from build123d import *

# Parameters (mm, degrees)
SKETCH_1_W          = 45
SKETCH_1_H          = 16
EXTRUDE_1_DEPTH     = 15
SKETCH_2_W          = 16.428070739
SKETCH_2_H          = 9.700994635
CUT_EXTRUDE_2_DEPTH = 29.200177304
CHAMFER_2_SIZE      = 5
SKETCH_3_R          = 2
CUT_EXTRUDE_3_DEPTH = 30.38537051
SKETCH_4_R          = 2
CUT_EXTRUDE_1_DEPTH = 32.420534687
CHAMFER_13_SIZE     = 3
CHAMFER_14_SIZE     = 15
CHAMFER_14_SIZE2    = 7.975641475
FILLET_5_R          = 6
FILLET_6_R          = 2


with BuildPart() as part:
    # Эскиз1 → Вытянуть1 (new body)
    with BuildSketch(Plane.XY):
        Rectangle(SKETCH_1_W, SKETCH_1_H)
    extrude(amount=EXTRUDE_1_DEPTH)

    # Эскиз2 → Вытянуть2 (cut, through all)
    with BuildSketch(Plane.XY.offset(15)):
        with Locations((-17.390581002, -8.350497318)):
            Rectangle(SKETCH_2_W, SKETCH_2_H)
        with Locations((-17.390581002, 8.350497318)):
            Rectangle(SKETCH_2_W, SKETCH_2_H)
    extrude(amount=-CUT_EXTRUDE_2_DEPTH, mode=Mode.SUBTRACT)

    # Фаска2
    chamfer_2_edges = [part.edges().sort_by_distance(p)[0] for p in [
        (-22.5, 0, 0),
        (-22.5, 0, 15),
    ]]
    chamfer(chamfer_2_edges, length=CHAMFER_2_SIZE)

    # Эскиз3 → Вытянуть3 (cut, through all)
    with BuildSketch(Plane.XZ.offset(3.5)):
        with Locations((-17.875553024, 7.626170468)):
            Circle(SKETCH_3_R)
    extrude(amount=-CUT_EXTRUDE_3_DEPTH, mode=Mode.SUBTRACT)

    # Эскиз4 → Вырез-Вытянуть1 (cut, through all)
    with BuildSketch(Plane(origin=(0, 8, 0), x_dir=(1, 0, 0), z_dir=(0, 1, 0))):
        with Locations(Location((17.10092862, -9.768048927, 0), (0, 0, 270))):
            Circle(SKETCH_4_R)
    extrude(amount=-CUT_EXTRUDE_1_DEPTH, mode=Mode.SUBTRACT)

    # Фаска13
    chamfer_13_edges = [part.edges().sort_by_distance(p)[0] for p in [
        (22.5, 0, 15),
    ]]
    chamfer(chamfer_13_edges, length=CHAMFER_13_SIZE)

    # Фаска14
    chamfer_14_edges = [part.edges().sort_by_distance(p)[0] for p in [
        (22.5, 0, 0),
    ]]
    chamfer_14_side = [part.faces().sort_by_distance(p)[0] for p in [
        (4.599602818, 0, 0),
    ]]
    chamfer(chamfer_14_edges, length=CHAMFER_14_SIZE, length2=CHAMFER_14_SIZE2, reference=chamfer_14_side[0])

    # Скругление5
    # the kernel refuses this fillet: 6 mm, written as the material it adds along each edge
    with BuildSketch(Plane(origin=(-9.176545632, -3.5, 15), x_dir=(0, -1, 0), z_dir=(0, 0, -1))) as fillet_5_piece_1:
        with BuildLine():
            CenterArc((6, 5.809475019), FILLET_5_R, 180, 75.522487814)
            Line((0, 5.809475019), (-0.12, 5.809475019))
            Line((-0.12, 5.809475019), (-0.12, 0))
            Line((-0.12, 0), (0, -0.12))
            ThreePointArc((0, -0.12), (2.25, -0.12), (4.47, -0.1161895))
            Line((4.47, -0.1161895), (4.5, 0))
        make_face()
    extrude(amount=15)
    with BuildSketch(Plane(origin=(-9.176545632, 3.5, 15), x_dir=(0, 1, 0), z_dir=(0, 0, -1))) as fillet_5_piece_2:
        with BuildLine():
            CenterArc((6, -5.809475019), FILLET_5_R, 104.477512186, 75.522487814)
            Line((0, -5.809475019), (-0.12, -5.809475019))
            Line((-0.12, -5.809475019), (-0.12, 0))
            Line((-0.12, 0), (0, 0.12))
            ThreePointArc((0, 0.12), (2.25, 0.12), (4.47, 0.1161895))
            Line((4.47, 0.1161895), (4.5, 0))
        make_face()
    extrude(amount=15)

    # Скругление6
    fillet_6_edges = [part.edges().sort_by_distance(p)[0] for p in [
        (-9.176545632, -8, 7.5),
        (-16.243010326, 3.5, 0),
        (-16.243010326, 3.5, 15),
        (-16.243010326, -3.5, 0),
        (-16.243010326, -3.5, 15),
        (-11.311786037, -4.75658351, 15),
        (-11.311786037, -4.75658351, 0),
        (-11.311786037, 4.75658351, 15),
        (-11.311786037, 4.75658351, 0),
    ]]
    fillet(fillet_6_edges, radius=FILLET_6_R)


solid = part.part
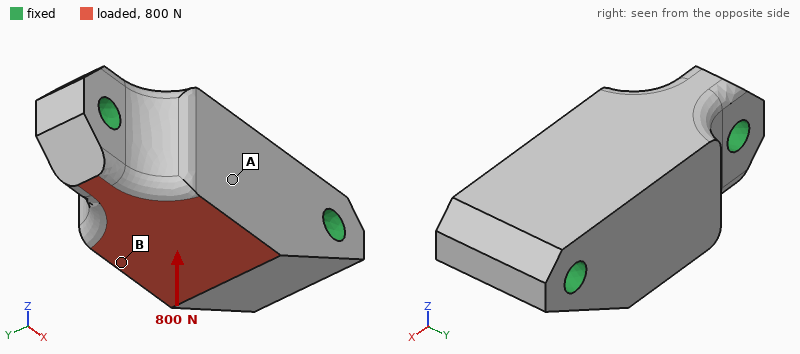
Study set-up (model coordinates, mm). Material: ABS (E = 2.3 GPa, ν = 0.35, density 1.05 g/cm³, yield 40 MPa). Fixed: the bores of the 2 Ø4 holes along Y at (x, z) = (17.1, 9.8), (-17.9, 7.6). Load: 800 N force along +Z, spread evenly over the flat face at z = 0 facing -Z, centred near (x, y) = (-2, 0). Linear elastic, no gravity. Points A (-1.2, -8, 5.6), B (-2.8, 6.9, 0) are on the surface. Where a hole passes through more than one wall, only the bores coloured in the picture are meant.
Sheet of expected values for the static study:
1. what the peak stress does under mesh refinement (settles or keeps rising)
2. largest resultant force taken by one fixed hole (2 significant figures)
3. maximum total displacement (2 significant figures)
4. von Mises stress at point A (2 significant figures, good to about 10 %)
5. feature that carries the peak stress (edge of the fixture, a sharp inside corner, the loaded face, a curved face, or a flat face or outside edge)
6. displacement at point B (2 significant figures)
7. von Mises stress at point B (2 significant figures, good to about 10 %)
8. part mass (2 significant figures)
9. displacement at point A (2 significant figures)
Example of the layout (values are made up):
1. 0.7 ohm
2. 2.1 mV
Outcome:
1. keeps rising
2. 430 N
3. 79 µm
4. 1.7 MPa
5. edge of the fixture
6. 77 µm
7. 5.4 MPa
8. 8.1 g
9. 74 µm
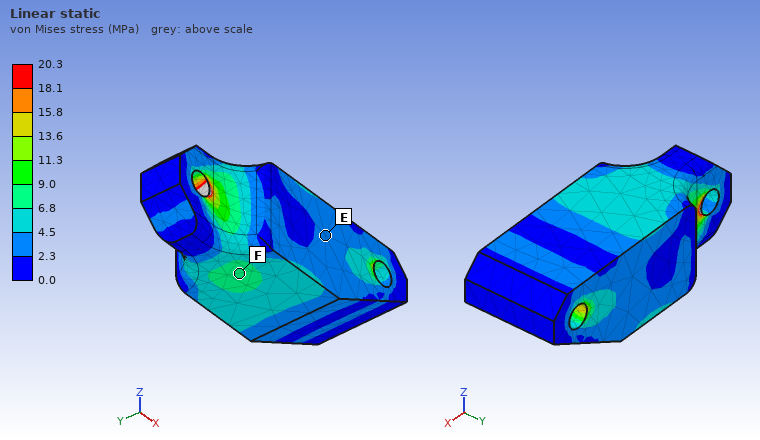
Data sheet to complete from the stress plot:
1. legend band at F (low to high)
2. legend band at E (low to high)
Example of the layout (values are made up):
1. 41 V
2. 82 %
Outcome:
1. 6.8 to 9.0 MPa
2. 2.3 to 4.5 MPa
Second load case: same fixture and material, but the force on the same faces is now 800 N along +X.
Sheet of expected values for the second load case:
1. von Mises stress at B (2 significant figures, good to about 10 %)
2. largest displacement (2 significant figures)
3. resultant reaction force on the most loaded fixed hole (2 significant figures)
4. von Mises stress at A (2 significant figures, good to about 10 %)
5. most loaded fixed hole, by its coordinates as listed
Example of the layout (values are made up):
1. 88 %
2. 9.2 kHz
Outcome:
1. 4.8 MPa
2. 35 µm
3. 490 N
4. 1.3 MPa
5. (17.1, 9.8)
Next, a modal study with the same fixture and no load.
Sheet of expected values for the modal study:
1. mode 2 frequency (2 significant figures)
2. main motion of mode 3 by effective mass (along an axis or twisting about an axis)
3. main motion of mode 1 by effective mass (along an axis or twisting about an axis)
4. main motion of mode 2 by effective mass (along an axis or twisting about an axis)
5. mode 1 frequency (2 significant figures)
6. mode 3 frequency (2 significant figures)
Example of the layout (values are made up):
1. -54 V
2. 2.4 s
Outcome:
1. 7900 Hz
2. along Y
3. along Z
4. along Y
5. 7500 Hz
6. 8800 Hz
